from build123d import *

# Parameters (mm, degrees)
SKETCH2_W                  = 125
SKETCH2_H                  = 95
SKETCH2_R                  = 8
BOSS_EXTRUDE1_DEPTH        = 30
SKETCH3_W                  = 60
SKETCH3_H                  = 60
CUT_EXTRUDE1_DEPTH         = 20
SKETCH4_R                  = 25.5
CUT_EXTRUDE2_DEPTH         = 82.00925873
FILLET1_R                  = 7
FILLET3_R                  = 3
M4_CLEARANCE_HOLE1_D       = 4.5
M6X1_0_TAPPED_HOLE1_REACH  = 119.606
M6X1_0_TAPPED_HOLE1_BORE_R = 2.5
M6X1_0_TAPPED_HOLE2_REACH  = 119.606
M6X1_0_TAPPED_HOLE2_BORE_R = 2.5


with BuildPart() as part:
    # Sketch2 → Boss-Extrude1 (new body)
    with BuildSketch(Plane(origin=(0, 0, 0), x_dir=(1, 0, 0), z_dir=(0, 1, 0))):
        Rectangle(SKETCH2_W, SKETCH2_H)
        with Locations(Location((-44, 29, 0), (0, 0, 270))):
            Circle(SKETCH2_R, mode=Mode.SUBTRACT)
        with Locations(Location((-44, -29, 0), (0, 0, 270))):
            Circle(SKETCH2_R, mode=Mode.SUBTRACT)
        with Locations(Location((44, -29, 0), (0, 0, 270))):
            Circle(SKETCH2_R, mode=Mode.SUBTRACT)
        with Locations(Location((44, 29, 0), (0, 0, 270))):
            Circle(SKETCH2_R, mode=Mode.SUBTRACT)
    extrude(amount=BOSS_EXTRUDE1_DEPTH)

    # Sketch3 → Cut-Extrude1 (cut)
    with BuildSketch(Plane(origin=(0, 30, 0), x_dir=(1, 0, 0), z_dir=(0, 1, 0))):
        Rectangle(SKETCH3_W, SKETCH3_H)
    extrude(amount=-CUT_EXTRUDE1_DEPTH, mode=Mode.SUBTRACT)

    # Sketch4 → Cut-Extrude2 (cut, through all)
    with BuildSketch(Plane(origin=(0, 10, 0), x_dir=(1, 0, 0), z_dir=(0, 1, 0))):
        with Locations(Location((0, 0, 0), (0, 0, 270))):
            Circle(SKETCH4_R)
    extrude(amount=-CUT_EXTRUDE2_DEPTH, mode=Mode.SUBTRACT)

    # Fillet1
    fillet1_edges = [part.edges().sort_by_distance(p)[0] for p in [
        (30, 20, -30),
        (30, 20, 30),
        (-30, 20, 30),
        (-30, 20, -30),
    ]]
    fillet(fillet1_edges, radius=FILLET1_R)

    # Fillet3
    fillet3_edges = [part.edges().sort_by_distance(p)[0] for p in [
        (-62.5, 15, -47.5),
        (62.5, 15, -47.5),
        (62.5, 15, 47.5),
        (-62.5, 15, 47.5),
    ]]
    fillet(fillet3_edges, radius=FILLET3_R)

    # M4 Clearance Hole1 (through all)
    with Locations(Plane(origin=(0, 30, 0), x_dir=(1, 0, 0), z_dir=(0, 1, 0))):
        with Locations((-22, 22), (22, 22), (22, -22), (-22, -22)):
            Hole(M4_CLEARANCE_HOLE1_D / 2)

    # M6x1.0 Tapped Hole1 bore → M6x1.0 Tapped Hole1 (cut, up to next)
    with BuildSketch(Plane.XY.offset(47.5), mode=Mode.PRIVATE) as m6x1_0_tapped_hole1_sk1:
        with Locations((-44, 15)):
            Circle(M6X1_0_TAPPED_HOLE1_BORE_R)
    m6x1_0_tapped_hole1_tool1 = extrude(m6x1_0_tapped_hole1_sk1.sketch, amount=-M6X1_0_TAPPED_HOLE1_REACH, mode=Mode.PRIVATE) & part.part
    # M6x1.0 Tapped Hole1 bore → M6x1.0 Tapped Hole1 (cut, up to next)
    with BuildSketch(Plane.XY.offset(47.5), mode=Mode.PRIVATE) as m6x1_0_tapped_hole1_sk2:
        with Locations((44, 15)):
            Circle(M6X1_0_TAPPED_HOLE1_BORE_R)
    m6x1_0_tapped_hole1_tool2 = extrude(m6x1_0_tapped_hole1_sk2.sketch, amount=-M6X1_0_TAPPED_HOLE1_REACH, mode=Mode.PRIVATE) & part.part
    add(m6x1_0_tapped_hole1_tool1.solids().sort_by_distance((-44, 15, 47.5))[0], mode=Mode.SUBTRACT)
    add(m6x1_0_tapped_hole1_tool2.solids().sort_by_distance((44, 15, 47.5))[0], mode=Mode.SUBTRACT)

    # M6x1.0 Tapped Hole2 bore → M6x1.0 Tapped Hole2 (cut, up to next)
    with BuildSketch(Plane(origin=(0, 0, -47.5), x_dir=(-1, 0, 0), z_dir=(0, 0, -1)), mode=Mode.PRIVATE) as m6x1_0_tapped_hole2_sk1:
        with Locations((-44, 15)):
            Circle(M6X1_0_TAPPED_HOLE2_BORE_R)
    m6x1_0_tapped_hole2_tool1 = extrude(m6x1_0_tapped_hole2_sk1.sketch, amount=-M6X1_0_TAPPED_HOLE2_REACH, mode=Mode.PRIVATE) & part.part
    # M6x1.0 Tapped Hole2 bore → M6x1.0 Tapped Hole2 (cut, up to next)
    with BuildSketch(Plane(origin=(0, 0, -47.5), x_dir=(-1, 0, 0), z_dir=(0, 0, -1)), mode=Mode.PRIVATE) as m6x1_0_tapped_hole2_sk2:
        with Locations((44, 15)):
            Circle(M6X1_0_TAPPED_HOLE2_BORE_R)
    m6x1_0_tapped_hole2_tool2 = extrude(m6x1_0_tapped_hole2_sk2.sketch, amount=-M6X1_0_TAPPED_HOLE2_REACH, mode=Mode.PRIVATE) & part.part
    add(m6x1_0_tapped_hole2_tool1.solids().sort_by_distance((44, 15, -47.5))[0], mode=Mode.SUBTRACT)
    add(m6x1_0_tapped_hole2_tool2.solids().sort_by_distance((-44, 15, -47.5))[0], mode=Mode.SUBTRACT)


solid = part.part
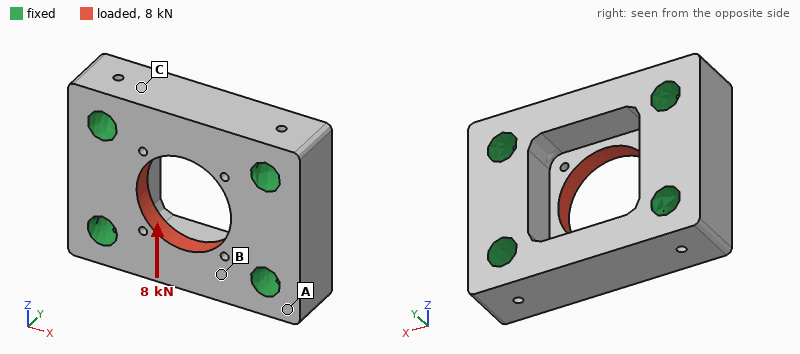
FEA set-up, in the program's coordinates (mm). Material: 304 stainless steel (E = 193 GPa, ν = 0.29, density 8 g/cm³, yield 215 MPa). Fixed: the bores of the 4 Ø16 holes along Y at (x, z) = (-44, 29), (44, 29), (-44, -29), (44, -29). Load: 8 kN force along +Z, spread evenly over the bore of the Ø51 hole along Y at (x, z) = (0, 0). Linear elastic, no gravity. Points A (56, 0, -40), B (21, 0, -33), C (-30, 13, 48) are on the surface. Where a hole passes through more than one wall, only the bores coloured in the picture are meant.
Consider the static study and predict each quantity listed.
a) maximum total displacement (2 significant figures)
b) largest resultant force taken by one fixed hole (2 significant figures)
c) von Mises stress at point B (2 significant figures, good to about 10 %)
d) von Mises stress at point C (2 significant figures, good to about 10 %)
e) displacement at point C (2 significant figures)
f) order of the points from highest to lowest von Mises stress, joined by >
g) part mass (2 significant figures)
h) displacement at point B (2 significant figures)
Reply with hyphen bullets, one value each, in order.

- 2.4 µm
- 2.1 kN
- 8.2 MPa
- 3.4 MPa
- 0.52 µm
- B > C > A
- 1.9 kg
- 1.1 µm
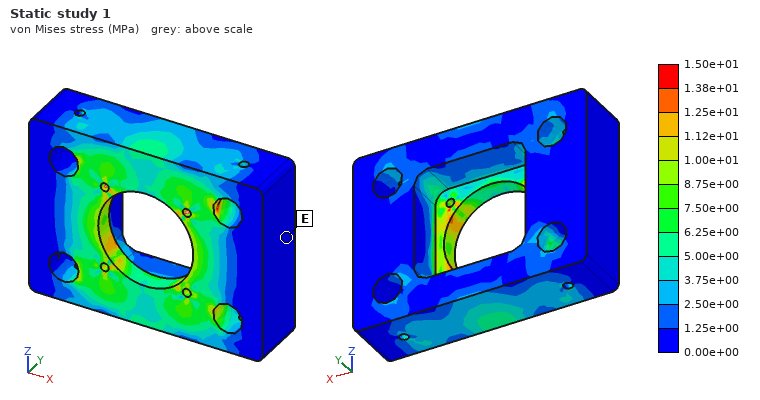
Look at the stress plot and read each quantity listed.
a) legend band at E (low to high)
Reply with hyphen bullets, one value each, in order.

- 0.00e+00 to 1.25e+00 MPa
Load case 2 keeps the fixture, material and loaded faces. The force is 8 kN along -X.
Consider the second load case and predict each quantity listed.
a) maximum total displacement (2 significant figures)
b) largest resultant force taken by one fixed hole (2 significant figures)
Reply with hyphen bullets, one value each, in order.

- 0.96 µm
- 2.1 kN
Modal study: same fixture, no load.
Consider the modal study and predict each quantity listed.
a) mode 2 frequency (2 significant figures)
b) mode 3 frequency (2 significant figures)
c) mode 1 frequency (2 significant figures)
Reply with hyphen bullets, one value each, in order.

- 15 kHz
- 15 kHz
- 15 kHz
